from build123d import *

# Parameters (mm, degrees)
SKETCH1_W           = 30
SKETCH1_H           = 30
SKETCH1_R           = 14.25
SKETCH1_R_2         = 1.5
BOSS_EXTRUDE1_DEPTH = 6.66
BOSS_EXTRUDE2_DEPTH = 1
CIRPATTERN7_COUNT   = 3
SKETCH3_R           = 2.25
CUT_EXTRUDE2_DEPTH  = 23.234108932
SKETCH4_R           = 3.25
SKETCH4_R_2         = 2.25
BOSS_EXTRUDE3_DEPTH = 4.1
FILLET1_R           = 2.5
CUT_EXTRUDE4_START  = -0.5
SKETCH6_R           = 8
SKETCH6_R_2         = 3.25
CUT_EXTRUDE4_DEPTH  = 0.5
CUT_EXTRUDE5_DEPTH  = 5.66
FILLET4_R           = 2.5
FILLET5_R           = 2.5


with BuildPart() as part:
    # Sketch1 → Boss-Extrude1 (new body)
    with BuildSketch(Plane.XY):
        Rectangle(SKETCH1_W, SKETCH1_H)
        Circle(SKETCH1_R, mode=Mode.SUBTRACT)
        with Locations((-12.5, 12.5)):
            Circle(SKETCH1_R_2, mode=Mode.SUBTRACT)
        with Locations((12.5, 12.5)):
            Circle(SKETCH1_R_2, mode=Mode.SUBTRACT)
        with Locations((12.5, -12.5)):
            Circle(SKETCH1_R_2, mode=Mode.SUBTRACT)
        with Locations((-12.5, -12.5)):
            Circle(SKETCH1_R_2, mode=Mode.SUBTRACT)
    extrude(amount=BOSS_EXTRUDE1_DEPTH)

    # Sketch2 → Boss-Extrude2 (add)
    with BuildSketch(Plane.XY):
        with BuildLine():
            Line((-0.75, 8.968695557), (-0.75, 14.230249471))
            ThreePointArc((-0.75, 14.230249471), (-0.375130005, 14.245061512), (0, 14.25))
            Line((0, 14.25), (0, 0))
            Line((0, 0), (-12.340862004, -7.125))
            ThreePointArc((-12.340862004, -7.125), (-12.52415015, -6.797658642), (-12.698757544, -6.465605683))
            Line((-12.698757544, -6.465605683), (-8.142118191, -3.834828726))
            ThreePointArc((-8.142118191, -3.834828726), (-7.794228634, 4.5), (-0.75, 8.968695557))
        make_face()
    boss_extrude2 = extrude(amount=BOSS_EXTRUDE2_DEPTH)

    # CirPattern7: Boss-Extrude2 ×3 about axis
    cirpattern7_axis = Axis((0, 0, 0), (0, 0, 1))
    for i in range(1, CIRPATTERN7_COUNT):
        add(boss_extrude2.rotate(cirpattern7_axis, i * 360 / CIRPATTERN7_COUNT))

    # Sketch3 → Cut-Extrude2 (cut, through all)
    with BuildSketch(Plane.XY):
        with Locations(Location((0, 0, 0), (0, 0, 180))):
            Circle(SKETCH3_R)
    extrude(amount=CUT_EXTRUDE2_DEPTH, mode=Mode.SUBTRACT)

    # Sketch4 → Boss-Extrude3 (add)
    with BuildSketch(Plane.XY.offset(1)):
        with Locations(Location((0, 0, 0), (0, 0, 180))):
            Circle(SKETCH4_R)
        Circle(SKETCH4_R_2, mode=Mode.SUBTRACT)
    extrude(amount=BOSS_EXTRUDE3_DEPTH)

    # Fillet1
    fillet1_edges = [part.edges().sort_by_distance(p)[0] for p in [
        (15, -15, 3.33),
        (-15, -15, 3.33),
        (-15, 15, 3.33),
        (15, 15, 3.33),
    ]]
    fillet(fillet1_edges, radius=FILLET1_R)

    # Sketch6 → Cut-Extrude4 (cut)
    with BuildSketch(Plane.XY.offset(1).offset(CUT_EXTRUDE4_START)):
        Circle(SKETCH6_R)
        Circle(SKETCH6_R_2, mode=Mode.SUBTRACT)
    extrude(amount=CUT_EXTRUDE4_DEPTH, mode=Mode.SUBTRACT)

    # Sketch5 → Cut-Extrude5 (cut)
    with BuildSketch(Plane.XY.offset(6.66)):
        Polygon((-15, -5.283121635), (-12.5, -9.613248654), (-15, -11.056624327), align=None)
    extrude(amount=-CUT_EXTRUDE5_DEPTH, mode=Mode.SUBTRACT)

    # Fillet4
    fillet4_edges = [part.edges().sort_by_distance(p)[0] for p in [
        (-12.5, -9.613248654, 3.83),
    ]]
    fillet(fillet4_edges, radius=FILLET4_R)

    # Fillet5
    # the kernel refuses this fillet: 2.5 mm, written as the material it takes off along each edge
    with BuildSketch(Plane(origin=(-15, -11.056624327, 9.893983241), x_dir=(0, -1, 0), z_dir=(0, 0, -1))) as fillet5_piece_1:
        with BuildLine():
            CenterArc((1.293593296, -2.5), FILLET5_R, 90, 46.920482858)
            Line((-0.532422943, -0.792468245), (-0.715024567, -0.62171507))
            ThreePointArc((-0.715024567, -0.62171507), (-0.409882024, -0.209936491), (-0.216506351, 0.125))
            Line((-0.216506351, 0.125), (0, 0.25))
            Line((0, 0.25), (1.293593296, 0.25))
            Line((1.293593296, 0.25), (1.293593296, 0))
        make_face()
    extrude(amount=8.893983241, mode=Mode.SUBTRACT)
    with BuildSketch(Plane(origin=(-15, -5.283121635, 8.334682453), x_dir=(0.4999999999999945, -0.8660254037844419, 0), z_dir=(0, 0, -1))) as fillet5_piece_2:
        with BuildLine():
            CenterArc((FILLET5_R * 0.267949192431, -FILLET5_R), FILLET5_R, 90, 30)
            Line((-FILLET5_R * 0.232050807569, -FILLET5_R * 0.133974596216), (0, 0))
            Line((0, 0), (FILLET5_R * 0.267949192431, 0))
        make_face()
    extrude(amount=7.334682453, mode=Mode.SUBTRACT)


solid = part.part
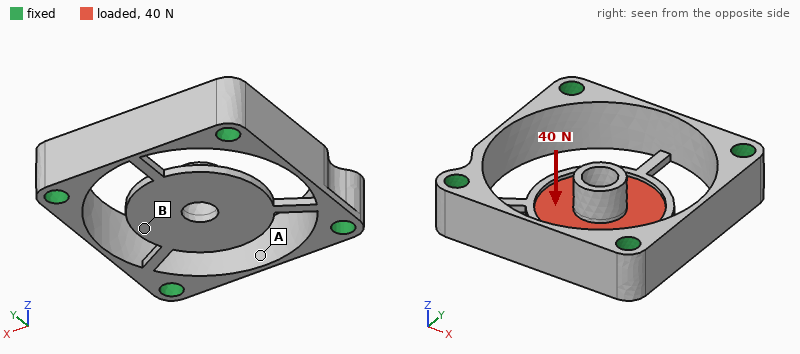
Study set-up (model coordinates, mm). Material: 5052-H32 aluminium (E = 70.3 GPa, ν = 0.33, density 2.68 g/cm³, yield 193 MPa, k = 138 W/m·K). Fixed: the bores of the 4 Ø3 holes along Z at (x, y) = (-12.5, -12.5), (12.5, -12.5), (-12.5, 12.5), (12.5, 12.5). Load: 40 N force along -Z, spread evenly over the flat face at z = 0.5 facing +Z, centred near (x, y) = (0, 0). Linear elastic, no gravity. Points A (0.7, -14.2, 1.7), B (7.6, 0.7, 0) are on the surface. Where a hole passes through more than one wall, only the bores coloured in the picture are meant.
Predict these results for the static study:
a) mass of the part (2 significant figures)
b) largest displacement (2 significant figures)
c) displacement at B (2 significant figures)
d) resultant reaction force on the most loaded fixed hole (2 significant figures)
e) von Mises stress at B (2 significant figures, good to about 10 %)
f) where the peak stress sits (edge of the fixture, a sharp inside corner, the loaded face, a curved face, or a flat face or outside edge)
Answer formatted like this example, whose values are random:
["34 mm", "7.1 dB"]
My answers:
["4.7 g", "0.13 mm", "0.11 mm", "29 N", "49 MPa", "a flat face or outside edge"]
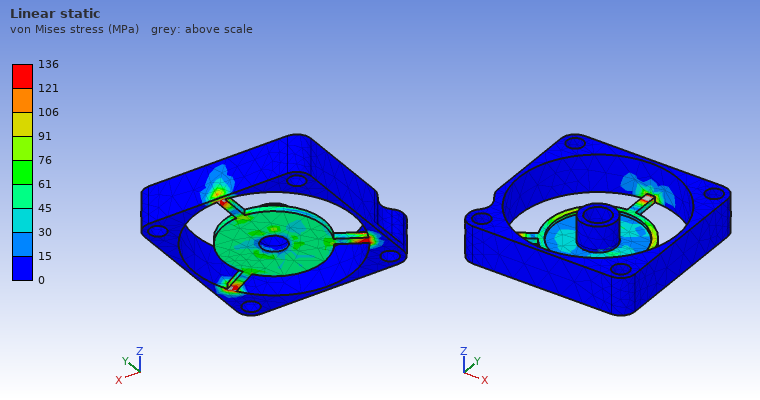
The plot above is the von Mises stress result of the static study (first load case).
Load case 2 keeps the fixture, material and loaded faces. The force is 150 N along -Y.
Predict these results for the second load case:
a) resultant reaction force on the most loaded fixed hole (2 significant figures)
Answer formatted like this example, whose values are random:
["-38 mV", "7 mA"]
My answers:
["78 N"]
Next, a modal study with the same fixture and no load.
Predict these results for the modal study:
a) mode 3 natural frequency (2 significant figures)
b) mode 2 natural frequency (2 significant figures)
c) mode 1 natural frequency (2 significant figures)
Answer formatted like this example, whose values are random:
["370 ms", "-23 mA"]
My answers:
["6000 Hz", "5800 Hz", "3700 Hz"]
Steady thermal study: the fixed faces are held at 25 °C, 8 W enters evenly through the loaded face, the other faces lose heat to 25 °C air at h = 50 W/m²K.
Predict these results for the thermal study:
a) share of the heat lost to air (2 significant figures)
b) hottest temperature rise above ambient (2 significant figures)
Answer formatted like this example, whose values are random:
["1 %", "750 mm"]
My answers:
["28 %", "77 K"]
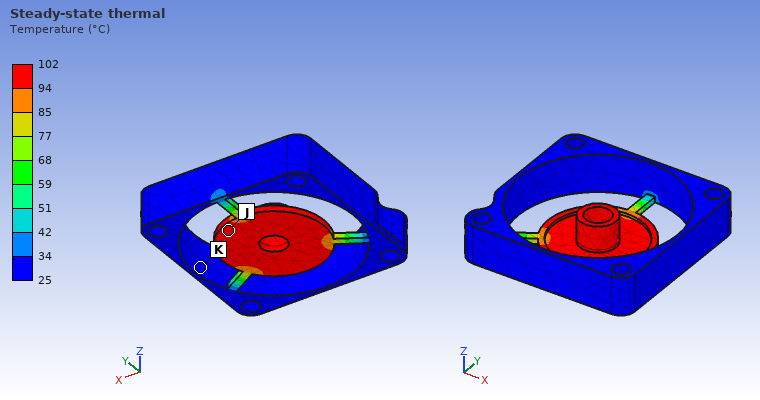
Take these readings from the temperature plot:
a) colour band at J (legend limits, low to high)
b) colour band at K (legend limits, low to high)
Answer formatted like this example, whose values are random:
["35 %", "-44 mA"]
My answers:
["94 to 102 °C", "25 to 34 °C"]
